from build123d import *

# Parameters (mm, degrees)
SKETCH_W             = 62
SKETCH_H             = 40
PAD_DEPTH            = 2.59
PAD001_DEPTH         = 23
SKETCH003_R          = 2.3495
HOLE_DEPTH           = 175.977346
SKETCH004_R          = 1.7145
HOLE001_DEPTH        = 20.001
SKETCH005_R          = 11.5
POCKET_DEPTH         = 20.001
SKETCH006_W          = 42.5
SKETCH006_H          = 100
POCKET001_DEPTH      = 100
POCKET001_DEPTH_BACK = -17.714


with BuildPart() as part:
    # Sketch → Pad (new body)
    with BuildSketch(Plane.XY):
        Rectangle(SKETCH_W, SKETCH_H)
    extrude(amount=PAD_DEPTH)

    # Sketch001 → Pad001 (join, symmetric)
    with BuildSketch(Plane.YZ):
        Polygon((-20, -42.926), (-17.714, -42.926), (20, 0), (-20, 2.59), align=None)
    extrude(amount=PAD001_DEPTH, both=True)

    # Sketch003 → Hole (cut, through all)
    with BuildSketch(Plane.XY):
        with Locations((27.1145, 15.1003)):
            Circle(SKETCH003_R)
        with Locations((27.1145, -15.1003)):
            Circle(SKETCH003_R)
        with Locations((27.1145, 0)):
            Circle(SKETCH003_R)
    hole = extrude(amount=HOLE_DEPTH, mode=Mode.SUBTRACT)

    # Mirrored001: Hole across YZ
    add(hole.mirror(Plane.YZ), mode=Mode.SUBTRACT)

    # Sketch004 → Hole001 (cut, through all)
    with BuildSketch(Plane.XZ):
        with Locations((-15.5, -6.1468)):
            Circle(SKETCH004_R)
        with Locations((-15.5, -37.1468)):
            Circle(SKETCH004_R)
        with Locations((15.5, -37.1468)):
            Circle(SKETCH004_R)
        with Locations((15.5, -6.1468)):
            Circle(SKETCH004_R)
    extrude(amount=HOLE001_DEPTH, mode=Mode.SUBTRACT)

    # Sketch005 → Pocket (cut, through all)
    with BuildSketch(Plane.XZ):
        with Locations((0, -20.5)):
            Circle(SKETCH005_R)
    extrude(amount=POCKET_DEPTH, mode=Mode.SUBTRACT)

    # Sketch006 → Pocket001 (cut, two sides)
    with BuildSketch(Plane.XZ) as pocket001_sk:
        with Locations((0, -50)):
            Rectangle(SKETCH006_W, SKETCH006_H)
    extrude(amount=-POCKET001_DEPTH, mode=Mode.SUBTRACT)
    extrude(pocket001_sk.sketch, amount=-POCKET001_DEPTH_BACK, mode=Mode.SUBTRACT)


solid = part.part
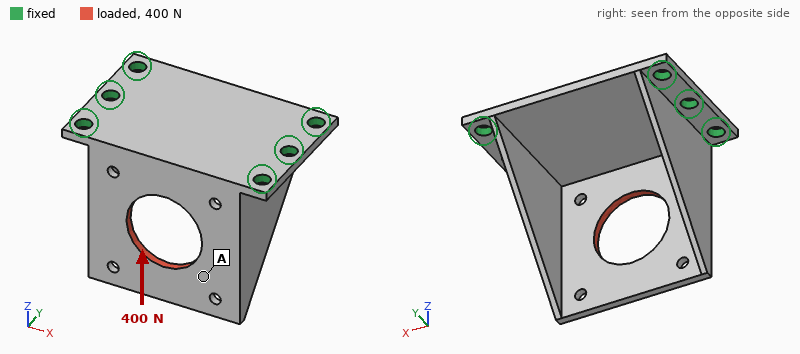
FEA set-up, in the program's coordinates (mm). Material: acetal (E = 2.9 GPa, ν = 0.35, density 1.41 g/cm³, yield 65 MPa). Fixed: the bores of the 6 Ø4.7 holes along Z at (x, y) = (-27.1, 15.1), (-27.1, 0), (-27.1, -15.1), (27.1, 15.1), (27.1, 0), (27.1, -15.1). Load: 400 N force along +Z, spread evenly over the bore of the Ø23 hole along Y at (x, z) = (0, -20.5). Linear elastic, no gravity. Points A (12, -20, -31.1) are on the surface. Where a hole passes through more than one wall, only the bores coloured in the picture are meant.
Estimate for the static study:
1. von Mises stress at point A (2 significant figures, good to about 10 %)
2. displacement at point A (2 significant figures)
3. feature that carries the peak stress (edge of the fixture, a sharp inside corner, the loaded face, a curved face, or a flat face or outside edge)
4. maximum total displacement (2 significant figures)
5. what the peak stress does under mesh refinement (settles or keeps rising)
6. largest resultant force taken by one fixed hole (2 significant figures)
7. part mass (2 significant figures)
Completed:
3.5 MPa
0.24 mm
edge of the fixture
0.32 mm
keeps rising
220 N
18 g
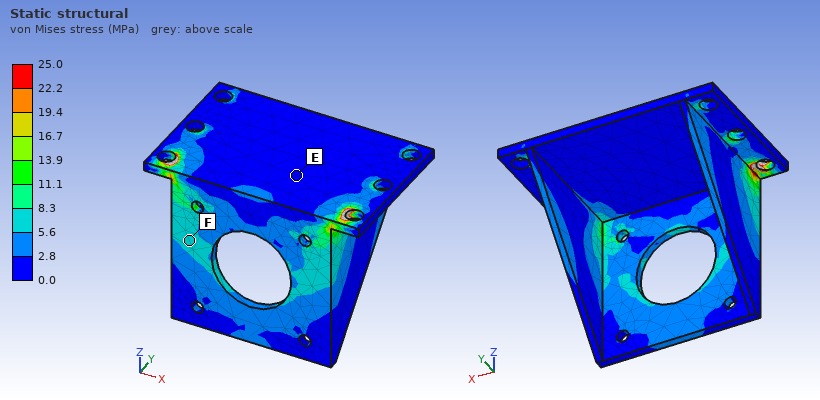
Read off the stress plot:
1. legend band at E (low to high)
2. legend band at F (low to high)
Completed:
0.0 to 2.8 MPa
5.6 to 8.3 MPa
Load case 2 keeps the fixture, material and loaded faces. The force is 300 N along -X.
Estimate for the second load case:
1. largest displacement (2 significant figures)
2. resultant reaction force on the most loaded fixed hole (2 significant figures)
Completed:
0.33 mm
180 N
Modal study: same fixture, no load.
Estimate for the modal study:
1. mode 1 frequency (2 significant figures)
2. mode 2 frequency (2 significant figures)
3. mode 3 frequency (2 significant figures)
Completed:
950 Hz
1600 Hz
1600 Hz
